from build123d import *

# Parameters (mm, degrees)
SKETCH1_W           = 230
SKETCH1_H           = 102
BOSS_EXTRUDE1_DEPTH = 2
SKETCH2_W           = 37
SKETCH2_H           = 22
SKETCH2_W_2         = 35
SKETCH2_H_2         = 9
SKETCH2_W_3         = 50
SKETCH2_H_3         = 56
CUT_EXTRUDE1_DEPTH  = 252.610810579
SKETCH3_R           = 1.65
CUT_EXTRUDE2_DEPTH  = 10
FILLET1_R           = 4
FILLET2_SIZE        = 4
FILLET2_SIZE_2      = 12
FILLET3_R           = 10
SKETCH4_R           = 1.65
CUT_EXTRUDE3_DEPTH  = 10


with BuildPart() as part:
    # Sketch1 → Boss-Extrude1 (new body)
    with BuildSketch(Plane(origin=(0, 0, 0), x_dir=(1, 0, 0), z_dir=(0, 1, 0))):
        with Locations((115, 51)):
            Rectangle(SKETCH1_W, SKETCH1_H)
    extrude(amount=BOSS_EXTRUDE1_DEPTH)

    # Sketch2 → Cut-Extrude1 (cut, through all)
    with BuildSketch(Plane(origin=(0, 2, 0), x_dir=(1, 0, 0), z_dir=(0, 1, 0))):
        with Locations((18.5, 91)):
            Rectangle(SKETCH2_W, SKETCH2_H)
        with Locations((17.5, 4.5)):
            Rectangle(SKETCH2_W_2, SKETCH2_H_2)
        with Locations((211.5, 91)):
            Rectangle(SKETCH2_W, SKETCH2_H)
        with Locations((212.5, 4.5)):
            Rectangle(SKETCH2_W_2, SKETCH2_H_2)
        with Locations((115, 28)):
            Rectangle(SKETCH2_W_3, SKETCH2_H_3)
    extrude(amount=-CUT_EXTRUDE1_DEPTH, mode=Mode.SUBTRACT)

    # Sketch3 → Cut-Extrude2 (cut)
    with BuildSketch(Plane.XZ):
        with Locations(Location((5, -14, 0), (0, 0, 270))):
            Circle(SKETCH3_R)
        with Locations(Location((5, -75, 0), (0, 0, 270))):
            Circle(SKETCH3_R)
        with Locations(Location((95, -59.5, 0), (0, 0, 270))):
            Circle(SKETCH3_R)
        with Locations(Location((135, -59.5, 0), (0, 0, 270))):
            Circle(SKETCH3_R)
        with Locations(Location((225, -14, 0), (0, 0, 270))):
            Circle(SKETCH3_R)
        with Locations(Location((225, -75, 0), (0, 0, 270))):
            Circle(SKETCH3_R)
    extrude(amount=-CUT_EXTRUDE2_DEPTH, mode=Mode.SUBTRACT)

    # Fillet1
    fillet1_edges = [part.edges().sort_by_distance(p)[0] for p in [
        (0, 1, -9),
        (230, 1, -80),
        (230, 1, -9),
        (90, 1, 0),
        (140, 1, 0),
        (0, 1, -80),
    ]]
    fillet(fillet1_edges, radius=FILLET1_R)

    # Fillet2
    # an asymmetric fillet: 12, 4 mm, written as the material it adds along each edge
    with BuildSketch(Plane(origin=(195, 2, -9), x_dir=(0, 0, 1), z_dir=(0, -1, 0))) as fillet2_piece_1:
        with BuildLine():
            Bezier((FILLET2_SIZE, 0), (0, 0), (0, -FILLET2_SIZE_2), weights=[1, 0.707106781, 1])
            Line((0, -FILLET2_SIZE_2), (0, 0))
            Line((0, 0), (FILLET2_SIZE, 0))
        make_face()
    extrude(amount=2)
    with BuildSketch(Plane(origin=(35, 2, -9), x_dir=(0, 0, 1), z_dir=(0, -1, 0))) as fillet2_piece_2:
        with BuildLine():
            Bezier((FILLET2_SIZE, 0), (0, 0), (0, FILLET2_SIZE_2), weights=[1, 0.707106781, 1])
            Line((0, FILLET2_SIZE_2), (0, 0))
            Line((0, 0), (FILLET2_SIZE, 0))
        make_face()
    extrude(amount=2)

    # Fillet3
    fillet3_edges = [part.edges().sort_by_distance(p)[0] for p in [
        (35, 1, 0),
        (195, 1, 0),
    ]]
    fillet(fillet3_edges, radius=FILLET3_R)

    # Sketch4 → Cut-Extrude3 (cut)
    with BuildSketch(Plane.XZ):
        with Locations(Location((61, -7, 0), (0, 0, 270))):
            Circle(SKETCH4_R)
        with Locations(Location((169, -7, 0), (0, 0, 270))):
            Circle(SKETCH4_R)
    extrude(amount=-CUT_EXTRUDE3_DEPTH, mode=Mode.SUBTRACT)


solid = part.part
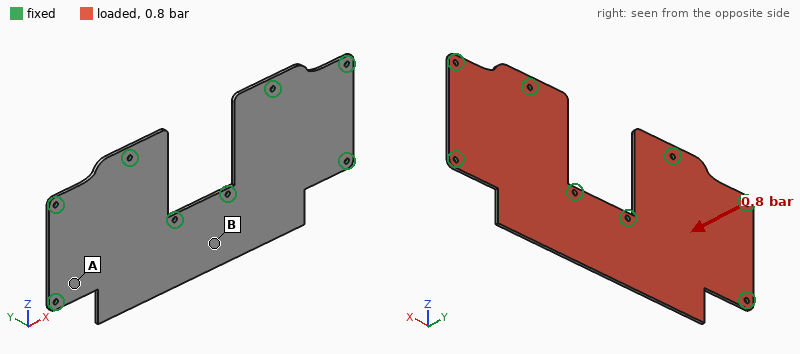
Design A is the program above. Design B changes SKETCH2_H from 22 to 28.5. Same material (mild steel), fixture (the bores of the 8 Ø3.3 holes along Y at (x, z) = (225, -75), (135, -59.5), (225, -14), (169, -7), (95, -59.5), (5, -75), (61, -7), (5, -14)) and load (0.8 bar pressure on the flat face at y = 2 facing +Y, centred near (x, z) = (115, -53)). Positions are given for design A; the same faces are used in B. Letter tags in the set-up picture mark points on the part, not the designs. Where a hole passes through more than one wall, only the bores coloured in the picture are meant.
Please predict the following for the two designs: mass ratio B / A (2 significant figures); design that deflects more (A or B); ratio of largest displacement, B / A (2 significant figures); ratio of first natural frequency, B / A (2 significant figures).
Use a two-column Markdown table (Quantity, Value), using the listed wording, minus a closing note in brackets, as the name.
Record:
| Quantity | Value |
|---|---|
| mass ratio B / A | 0.99 |
| design that deflects more | B |
| ratio of largest displacement, B / A | 1.1 |
| ratio of first natural frequency, B / A | 0.97 |
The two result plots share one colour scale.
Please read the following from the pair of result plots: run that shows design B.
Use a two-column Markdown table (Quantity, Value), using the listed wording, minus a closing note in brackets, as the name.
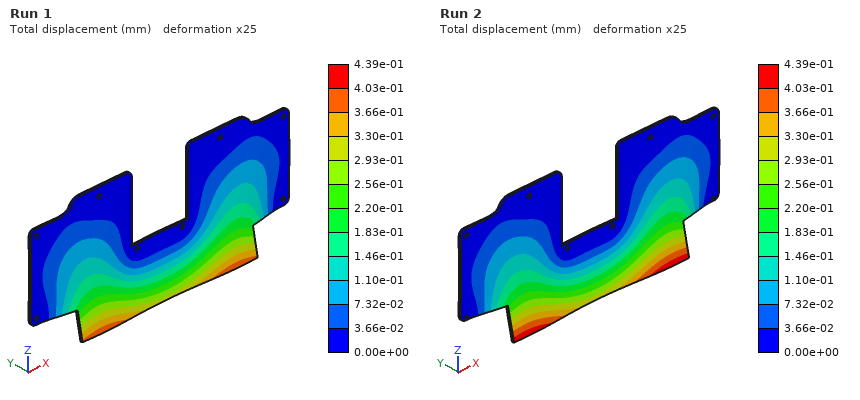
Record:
| Quantity | Value |
|---|---|
| run that shows design B | Run 2 |
